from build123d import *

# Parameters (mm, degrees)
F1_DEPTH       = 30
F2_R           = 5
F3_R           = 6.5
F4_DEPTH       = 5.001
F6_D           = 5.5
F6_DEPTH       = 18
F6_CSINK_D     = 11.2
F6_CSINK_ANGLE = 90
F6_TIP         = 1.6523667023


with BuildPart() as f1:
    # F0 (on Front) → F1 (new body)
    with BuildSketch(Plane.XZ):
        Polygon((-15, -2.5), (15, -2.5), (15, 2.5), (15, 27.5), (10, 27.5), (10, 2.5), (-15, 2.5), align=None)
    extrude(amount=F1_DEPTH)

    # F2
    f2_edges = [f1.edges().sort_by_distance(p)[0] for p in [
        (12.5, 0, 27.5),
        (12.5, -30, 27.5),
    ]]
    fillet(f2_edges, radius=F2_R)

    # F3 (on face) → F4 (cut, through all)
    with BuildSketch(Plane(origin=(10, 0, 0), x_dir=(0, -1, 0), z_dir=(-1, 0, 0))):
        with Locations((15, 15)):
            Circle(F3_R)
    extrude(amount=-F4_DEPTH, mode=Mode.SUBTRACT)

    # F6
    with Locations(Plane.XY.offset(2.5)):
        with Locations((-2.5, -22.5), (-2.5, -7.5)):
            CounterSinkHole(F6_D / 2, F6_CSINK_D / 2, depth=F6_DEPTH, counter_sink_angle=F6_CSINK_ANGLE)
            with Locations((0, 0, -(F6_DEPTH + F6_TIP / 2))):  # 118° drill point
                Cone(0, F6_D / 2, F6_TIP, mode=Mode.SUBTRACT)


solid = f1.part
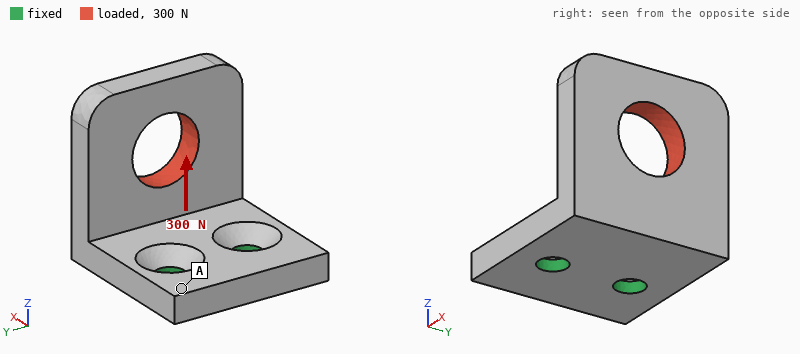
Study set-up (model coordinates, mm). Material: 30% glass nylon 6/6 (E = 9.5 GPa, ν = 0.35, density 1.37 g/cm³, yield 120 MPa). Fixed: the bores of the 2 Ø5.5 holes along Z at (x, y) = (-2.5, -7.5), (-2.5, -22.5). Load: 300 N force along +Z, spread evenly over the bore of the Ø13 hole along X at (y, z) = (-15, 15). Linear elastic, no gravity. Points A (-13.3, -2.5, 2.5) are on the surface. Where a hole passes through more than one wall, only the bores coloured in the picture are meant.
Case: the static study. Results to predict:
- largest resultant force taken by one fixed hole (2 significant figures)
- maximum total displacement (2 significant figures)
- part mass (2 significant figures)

150 N
0.55 mm
9.7 g
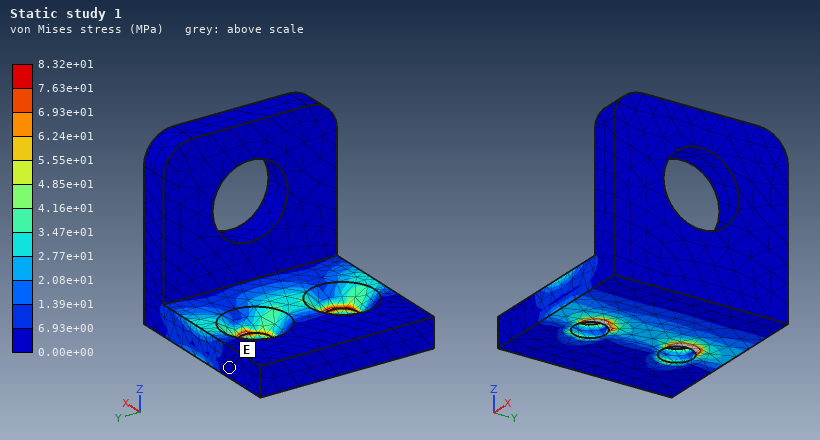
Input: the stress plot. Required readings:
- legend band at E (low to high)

0.00e+00 to 6.93e+00 MPa
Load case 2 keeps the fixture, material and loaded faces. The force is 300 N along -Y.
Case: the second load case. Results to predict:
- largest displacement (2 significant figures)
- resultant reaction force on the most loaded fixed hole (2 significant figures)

0.31 mm
410 N
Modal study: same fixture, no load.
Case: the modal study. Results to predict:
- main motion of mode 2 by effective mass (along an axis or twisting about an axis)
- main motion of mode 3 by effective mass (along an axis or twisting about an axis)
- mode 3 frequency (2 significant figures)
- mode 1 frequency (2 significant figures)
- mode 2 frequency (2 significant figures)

along Y
along Z
4300 Hz
1400 Hz
2600 Hz
